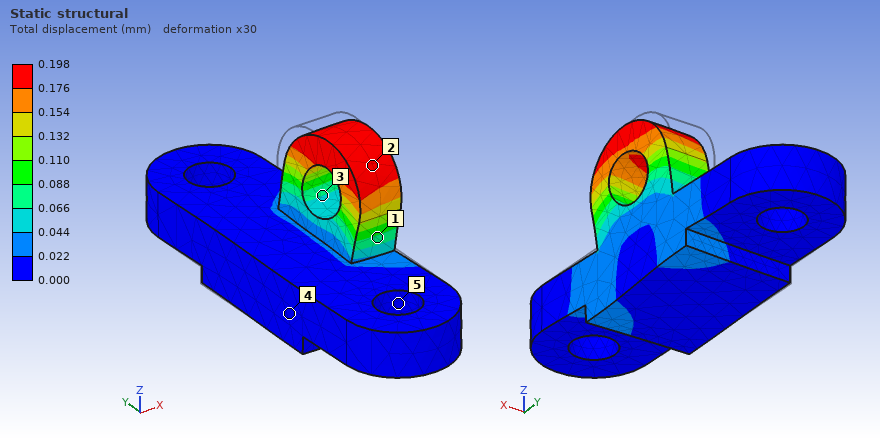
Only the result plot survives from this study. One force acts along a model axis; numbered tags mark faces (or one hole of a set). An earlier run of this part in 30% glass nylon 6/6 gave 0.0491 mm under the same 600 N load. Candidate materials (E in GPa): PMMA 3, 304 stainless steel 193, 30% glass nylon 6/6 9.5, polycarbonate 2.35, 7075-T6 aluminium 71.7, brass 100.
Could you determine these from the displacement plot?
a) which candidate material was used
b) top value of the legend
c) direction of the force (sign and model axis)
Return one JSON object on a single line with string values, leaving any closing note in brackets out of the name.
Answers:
{"which candidate material was used": "polycarbonate", "top value of the legend": "0.198 mm", "direction of the force": "-Y"}
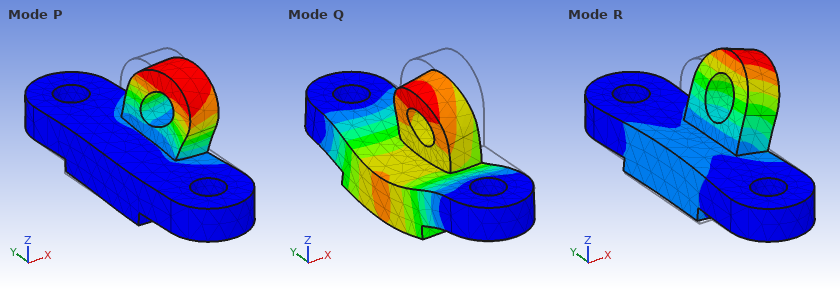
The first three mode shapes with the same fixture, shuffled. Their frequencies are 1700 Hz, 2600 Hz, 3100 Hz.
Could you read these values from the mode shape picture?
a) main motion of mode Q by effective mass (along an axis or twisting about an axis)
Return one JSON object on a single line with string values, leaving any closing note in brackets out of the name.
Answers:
{"main motion of mode Q by effective mass": "along Z"}
